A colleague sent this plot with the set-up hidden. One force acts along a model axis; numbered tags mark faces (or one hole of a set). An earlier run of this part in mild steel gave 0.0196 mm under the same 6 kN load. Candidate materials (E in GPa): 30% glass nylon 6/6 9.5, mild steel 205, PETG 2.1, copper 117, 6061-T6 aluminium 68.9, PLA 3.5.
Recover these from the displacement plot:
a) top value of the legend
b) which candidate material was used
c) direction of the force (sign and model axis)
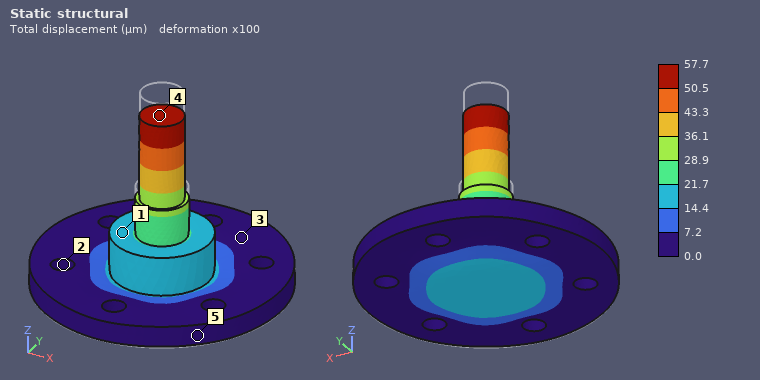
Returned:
57.7 µm
6061-T6 aluminium
-Z
